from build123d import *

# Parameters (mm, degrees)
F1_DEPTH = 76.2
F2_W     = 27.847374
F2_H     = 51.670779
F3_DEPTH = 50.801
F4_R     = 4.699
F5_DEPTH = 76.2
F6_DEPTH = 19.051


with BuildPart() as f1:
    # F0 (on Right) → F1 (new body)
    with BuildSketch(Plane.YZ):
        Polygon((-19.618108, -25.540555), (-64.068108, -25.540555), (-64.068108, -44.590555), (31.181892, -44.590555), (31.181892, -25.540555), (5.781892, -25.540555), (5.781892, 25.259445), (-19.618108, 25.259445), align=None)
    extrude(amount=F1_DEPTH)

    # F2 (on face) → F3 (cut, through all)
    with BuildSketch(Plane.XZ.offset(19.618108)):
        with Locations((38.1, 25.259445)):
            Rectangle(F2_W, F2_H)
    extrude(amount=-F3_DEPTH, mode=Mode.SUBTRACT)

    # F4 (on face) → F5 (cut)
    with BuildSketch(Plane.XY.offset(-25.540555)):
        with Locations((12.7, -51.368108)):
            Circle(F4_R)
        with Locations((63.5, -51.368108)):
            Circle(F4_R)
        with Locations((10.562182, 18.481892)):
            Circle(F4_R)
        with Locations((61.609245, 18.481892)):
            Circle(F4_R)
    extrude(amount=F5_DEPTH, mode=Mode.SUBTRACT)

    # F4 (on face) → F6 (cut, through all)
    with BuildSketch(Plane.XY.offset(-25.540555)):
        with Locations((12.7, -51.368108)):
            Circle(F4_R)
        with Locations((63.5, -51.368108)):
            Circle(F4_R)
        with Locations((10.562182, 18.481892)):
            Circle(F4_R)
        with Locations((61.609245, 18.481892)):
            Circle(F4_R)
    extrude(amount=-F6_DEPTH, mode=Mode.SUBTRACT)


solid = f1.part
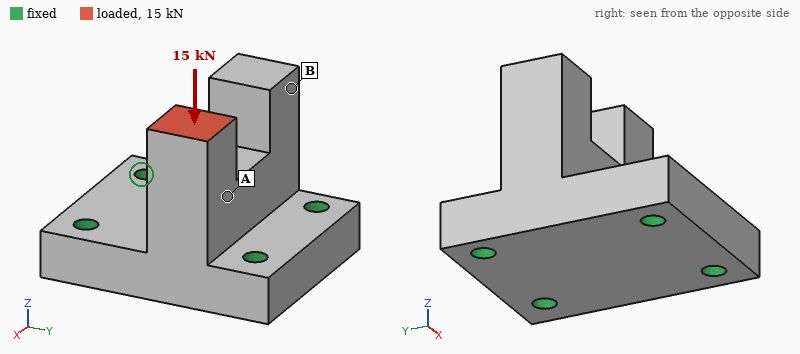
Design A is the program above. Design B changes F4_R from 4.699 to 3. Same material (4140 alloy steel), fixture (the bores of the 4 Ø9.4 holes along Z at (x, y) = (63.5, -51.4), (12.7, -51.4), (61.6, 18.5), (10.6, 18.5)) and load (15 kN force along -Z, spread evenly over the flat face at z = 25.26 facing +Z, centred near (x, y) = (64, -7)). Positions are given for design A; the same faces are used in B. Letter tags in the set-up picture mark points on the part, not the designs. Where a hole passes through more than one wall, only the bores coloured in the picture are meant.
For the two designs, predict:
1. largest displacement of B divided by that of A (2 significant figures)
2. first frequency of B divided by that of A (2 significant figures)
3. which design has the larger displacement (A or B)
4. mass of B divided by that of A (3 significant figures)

1.1
0.97
B
1.01
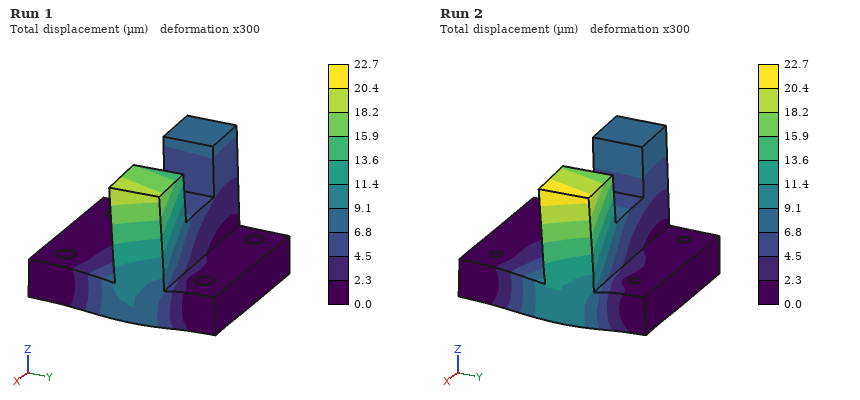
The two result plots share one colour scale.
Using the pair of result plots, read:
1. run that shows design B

Run 2
